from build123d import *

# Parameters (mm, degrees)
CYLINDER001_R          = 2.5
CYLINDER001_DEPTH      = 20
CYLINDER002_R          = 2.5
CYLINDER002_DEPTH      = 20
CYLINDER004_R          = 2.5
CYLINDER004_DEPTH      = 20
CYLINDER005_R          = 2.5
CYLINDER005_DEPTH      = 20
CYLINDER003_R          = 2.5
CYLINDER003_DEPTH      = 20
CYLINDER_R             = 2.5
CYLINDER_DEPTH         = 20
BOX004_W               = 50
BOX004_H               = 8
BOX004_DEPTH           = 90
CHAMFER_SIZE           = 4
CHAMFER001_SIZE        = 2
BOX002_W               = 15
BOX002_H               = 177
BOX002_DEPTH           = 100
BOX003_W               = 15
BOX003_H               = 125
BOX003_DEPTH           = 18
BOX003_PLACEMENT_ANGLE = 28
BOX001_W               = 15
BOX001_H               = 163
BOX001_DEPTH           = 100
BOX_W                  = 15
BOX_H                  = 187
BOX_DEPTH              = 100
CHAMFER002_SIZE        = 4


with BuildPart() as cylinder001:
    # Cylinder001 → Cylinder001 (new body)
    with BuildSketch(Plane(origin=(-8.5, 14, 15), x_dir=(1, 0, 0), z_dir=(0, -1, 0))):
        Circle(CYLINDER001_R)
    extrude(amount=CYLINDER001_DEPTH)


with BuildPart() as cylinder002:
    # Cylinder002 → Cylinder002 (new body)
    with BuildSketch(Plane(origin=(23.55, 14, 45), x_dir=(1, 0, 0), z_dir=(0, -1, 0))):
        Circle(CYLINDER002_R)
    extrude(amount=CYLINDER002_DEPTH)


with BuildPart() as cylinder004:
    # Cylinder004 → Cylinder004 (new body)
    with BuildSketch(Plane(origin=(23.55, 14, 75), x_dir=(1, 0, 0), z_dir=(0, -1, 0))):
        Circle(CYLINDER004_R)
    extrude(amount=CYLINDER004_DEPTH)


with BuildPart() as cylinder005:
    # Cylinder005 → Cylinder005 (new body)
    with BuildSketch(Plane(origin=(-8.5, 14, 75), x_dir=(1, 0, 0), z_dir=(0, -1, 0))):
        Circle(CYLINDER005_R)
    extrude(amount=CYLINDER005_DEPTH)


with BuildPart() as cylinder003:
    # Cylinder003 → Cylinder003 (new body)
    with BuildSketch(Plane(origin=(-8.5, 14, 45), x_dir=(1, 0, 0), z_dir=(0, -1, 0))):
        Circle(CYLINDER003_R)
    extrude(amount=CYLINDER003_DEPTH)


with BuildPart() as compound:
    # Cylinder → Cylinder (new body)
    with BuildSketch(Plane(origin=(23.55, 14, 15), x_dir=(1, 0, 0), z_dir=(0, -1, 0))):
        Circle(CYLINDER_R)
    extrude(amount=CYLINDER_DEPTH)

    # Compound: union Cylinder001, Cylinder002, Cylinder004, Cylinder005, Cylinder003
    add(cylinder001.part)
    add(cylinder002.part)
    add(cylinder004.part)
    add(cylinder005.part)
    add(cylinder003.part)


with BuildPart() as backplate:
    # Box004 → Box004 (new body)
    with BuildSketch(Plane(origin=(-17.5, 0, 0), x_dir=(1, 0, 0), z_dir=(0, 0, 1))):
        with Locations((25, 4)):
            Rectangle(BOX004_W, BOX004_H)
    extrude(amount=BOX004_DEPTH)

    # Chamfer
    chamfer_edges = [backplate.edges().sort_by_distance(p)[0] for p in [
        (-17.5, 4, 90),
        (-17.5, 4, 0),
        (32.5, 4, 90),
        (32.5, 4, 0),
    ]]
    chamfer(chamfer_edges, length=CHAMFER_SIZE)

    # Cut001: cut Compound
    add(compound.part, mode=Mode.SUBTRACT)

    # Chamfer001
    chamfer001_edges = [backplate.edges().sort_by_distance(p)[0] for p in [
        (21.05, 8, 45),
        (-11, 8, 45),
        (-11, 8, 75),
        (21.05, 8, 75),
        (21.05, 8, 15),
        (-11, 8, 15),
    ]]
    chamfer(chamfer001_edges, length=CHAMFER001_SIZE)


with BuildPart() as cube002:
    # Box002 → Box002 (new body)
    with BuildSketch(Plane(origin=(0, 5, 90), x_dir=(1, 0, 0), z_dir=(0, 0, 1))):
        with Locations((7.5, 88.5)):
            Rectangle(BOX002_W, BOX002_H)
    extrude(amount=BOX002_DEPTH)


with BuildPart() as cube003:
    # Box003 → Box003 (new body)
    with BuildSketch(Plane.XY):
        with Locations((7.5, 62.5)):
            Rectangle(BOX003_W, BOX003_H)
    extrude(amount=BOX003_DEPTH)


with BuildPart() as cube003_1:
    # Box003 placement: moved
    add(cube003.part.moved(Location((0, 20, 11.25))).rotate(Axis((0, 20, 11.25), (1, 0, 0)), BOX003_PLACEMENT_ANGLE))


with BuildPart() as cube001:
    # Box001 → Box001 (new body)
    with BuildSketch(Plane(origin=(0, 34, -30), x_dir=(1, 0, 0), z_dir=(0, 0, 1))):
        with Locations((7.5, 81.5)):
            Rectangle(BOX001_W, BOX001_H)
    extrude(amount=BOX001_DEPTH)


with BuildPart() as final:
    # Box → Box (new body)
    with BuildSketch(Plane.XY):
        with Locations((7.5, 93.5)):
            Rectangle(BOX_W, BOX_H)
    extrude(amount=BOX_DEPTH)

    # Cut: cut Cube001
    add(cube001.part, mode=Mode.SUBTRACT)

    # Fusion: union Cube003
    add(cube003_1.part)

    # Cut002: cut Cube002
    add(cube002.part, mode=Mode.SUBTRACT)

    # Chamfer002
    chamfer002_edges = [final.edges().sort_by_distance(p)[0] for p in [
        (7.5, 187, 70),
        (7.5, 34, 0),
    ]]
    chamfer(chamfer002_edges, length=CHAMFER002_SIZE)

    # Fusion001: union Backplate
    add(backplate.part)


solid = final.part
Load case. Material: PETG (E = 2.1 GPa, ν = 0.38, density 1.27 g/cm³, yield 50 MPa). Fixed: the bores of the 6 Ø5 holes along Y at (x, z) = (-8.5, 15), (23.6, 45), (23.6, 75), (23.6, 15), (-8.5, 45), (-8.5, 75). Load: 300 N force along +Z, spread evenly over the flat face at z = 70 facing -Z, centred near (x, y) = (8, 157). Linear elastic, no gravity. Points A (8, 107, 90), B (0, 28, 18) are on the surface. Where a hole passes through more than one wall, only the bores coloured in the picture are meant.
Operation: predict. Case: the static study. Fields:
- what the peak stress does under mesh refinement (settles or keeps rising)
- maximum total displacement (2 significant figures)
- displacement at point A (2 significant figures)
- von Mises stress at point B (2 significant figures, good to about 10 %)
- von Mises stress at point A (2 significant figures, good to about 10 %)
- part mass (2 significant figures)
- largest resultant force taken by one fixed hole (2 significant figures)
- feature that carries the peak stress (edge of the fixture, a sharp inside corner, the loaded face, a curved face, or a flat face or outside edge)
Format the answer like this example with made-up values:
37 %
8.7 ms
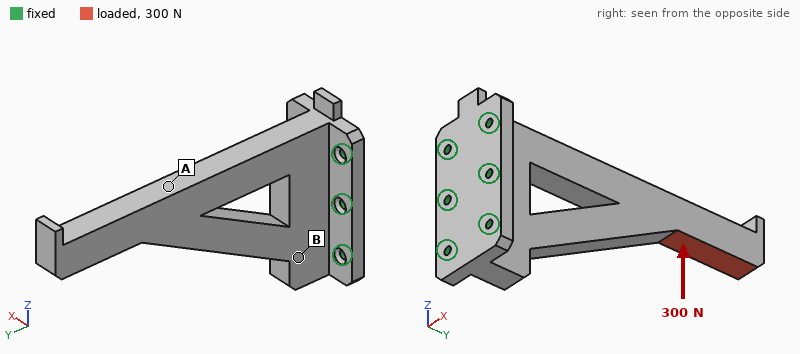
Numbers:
keeps rising
2.3 mm
0.62 mm
2.4 MPa
6.4 MPa
180 g
410 N
edge of the fixture
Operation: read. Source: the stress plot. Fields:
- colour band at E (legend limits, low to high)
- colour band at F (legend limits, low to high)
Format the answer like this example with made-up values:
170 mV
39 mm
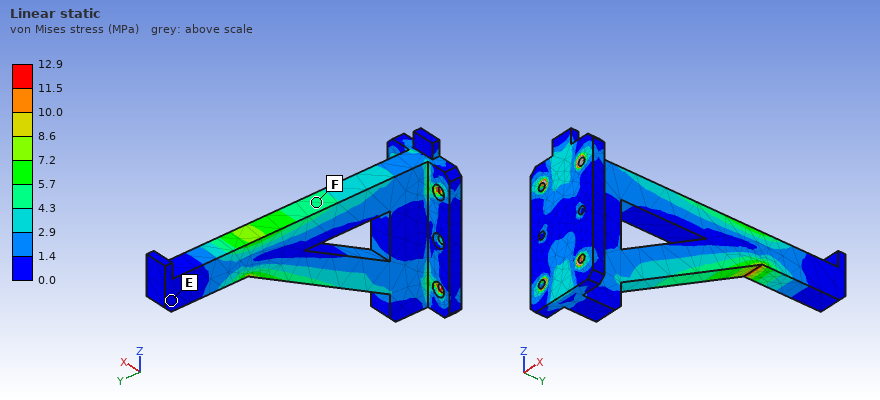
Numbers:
0.0 to 1.4 MPa
4.3 to 5.7 MPa
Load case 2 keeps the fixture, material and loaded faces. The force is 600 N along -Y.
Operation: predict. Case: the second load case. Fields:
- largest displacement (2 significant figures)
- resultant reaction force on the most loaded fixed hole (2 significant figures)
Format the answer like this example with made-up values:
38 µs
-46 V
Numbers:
0.38 mm
250 N
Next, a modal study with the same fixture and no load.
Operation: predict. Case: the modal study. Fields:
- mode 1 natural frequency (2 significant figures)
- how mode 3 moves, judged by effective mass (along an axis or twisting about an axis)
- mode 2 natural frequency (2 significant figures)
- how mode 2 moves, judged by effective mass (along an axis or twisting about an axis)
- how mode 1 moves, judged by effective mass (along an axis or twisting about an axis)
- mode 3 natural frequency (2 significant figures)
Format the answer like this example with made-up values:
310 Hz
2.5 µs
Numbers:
130 Hz
along X
400 Hz
along Z
along X
580 Hz
